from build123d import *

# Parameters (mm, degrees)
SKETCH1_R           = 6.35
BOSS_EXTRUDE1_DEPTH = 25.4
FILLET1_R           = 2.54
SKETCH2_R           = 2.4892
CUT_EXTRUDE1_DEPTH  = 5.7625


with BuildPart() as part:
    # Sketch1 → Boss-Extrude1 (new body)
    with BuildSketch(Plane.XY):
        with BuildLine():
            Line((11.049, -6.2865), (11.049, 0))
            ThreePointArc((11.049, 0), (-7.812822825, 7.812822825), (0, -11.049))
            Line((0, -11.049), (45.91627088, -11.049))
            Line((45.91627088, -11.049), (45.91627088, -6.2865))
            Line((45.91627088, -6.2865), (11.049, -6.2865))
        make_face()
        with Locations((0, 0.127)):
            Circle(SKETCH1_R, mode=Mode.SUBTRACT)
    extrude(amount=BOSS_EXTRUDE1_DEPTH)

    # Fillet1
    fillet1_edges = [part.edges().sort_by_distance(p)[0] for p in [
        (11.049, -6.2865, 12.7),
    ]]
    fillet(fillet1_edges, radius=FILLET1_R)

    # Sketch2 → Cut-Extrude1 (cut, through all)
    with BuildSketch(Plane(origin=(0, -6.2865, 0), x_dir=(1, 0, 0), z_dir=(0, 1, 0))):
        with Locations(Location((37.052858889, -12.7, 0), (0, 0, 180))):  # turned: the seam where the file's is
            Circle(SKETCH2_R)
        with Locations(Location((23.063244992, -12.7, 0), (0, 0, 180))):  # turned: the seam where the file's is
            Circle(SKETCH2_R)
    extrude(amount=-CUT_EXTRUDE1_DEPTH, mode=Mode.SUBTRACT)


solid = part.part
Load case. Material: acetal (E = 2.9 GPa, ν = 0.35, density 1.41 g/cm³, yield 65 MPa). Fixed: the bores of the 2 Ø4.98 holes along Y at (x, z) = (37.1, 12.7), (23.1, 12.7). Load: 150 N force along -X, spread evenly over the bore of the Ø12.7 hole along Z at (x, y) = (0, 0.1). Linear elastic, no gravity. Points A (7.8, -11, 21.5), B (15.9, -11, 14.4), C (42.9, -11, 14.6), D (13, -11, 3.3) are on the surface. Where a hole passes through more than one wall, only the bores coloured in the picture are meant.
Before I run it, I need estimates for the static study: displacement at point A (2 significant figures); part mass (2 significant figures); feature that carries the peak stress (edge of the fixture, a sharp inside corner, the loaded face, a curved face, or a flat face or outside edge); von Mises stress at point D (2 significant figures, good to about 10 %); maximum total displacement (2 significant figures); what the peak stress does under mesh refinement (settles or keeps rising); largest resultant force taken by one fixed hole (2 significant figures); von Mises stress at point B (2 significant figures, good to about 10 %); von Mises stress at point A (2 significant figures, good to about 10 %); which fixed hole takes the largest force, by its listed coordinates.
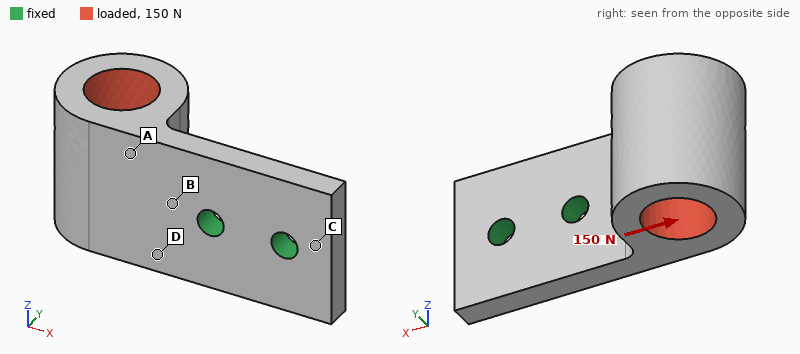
0.22 mm
16 g
edge of the fixture
10 MPa
0.76 mm
keeps rising
120 N
12 MPa
3.4 MPa
(23.1, 12.7)
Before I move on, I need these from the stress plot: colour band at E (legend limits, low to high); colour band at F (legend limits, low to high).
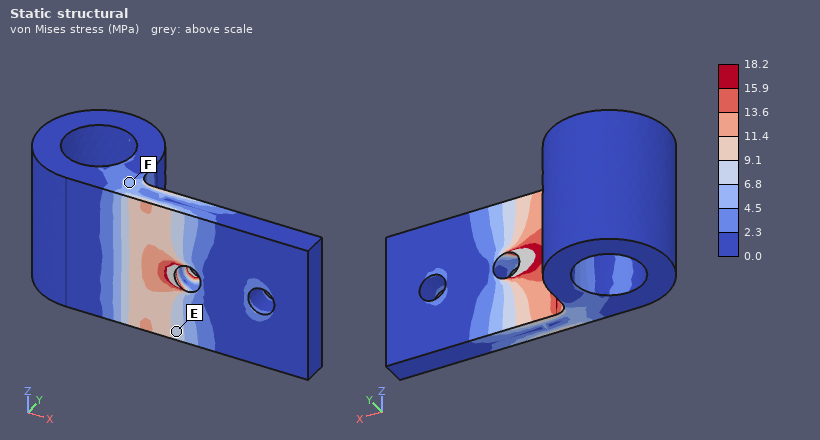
6.8 to 9.1 MPa
4.5 to 6.8 MPa
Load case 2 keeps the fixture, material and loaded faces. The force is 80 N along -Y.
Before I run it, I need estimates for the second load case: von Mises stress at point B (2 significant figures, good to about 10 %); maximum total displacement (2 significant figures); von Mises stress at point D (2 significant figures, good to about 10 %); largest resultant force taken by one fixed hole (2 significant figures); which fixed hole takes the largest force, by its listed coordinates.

14 MPa
0.78 mm
9.3 MPa
120 N
(23.1, 12.7)
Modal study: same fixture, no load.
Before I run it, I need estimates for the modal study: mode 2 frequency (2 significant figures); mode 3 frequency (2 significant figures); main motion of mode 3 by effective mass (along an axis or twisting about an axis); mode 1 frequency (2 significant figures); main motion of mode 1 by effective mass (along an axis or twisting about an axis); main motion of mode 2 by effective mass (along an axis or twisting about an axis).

1100 Hz
2300 Hz
along Z
560 Hz
along Y
along Z
